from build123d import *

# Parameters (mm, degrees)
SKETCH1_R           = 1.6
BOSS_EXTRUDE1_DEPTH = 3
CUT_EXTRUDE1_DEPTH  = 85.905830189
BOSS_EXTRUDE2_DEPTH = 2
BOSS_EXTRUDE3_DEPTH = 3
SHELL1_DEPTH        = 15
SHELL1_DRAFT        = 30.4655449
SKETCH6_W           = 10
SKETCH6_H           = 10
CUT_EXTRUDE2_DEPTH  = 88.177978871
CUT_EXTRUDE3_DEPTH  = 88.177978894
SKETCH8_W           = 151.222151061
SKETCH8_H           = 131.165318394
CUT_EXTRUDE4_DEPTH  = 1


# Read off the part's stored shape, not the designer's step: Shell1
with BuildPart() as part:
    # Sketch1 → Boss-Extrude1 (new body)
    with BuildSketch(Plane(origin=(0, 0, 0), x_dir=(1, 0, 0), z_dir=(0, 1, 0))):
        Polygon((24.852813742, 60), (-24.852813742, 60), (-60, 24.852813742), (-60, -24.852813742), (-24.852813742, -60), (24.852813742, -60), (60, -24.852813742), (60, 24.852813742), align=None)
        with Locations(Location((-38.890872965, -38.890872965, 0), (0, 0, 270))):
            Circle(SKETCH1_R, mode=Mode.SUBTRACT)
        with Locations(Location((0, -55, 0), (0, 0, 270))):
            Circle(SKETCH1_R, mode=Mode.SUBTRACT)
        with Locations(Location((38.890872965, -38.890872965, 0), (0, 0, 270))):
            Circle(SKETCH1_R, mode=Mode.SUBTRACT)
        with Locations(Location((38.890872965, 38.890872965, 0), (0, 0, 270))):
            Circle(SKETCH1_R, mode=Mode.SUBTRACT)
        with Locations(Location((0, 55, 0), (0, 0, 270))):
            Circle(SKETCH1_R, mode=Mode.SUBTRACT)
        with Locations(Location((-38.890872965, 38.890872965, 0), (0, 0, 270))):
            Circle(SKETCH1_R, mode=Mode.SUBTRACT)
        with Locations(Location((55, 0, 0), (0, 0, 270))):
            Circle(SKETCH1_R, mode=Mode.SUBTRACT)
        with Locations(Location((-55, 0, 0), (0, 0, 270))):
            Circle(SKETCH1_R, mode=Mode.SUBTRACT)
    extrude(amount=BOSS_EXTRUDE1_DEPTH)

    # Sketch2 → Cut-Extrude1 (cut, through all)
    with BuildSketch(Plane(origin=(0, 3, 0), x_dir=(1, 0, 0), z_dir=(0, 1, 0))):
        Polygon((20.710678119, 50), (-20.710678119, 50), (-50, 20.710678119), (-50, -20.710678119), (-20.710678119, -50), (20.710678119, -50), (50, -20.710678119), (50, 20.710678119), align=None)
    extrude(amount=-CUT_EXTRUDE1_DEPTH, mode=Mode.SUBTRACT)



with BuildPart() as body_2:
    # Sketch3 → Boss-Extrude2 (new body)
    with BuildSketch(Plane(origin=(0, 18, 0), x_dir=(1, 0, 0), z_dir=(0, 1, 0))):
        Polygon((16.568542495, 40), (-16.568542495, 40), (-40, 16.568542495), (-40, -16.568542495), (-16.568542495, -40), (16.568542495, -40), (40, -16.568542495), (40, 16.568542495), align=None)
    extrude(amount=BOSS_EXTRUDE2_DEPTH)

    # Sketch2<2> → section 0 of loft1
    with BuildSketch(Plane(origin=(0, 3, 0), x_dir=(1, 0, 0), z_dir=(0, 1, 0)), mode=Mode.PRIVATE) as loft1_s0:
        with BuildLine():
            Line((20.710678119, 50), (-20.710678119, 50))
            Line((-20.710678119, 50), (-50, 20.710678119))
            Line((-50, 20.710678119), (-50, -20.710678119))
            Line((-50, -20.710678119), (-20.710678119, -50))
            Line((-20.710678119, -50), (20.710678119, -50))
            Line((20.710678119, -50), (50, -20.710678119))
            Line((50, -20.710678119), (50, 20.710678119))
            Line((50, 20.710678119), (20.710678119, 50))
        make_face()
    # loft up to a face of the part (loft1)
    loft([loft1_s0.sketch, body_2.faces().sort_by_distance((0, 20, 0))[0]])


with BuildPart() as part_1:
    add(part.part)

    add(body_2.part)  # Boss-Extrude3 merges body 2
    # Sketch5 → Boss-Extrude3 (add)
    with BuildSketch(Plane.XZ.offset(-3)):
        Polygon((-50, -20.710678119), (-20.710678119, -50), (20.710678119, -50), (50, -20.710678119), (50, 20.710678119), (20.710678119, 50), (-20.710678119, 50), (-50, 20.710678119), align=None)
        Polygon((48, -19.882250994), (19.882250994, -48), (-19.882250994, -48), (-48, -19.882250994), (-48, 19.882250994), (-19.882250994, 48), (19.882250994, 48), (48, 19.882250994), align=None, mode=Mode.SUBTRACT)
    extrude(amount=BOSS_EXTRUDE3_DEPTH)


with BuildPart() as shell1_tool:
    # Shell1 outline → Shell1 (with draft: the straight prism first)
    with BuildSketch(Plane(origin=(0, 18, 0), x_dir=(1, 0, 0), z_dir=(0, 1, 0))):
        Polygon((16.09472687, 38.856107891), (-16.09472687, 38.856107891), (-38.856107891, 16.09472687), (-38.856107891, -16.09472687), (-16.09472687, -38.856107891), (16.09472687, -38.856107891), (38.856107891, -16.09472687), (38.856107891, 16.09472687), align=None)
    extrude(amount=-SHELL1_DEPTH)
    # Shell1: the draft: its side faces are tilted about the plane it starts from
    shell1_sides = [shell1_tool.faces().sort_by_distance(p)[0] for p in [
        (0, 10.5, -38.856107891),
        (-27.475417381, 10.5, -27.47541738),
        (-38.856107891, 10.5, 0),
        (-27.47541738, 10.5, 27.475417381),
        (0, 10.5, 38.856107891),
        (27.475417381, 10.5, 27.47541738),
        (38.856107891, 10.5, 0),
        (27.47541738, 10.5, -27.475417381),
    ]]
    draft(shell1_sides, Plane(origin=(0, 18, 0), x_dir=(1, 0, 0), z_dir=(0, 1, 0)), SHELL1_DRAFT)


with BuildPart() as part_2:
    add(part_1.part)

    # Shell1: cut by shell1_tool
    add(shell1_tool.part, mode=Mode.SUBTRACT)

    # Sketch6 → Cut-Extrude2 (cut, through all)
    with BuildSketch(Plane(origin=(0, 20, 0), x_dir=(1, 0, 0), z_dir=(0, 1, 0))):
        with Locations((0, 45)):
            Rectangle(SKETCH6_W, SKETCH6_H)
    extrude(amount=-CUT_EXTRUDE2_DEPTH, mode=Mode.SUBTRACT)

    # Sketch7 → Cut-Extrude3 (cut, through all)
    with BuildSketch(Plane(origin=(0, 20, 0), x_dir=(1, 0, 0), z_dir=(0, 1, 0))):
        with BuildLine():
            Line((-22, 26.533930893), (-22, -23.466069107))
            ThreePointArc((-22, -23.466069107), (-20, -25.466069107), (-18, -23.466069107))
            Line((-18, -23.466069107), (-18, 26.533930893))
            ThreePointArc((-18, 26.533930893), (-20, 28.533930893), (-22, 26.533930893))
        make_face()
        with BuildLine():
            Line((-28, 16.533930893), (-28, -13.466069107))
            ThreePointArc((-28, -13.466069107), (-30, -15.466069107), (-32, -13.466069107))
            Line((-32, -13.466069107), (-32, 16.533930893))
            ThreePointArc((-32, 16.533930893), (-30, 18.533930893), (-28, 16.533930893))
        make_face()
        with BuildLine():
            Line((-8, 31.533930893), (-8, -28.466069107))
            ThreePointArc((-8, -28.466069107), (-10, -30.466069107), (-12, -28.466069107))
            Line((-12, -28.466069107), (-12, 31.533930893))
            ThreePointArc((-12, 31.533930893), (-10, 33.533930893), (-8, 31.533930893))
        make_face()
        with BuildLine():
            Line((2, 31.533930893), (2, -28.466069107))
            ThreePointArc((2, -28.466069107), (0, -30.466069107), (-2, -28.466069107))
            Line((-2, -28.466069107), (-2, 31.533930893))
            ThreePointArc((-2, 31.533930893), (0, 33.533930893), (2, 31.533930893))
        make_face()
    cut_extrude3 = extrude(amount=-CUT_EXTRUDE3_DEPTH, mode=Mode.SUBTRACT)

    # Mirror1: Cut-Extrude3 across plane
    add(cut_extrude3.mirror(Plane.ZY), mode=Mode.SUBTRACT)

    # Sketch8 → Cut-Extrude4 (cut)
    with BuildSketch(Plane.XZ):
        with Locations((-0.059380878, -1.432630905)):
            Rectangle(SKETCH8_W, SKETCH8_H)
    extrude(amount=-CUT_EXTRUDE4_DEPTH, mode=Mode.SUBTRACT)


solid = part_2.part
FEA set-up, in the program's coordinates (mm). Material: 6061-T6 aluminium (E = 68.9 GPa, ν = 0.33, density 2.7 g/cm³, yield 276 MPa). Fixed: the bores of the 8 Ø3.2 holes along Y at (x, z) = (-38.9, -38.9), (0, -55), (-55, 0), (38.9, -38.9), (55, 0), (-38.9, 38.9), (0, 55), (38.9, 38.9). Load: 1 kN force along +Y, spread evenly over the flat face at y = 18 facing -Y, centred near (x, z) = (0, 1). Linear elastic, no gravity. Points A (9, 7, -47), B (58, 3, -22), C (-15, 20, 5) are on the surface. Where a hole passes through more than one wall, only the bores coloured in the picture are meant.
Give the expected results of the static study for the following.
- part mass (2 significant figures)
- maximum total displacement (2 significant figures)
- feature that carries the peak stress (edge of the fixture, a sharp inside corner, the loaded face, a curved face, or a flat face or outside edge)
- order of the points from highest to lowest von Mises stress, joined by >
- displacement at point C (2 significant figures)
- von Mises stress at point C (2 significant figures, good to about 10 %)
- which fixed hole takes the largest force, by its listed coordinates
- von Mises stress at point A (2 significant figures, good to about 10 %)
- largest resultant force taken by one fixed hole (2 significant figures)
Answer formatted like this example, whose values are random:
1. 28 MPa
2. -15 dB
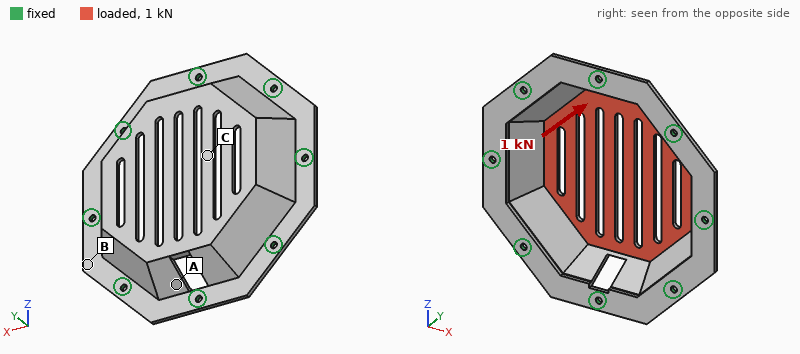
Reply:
1. 71 g
2. 0.62 mm
3. the loaded face
4. C > A > B
5. 0.37 mm
6. 77 MPa
7. (0, 55)
8. 20 MPa
9. 260 N
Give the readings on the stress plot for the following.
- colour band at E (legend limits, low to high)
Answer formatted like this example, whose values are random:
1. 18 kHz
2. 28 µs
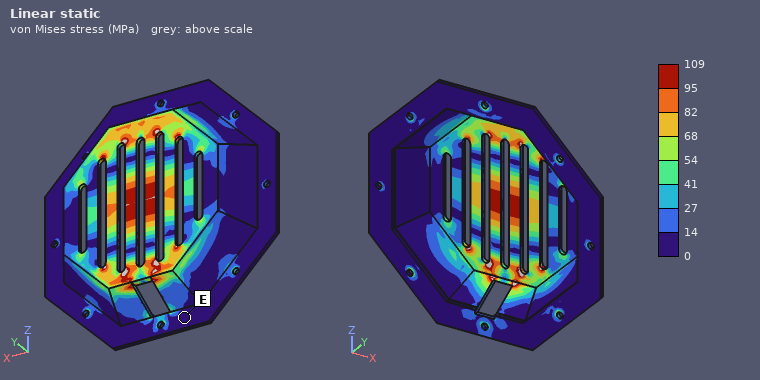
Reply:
1. 0 to 14 MPa
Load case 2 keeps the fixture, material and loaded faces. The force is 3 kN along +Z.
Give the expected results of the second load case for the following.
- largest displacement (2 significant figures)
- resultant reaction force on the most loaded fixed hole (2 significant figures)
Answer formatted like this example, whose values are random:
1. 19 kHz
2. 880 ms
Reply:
1. 68 µm
2. 490 N
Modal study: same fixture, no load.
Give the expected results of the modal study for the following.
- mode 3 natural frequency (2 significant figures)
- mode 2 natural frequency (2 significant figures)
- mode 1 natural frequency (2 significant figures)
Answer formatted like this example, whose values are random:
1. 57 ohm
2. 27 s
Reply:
1. 2400 Hz
2. 2100 Hz
3. 1800 Hz
